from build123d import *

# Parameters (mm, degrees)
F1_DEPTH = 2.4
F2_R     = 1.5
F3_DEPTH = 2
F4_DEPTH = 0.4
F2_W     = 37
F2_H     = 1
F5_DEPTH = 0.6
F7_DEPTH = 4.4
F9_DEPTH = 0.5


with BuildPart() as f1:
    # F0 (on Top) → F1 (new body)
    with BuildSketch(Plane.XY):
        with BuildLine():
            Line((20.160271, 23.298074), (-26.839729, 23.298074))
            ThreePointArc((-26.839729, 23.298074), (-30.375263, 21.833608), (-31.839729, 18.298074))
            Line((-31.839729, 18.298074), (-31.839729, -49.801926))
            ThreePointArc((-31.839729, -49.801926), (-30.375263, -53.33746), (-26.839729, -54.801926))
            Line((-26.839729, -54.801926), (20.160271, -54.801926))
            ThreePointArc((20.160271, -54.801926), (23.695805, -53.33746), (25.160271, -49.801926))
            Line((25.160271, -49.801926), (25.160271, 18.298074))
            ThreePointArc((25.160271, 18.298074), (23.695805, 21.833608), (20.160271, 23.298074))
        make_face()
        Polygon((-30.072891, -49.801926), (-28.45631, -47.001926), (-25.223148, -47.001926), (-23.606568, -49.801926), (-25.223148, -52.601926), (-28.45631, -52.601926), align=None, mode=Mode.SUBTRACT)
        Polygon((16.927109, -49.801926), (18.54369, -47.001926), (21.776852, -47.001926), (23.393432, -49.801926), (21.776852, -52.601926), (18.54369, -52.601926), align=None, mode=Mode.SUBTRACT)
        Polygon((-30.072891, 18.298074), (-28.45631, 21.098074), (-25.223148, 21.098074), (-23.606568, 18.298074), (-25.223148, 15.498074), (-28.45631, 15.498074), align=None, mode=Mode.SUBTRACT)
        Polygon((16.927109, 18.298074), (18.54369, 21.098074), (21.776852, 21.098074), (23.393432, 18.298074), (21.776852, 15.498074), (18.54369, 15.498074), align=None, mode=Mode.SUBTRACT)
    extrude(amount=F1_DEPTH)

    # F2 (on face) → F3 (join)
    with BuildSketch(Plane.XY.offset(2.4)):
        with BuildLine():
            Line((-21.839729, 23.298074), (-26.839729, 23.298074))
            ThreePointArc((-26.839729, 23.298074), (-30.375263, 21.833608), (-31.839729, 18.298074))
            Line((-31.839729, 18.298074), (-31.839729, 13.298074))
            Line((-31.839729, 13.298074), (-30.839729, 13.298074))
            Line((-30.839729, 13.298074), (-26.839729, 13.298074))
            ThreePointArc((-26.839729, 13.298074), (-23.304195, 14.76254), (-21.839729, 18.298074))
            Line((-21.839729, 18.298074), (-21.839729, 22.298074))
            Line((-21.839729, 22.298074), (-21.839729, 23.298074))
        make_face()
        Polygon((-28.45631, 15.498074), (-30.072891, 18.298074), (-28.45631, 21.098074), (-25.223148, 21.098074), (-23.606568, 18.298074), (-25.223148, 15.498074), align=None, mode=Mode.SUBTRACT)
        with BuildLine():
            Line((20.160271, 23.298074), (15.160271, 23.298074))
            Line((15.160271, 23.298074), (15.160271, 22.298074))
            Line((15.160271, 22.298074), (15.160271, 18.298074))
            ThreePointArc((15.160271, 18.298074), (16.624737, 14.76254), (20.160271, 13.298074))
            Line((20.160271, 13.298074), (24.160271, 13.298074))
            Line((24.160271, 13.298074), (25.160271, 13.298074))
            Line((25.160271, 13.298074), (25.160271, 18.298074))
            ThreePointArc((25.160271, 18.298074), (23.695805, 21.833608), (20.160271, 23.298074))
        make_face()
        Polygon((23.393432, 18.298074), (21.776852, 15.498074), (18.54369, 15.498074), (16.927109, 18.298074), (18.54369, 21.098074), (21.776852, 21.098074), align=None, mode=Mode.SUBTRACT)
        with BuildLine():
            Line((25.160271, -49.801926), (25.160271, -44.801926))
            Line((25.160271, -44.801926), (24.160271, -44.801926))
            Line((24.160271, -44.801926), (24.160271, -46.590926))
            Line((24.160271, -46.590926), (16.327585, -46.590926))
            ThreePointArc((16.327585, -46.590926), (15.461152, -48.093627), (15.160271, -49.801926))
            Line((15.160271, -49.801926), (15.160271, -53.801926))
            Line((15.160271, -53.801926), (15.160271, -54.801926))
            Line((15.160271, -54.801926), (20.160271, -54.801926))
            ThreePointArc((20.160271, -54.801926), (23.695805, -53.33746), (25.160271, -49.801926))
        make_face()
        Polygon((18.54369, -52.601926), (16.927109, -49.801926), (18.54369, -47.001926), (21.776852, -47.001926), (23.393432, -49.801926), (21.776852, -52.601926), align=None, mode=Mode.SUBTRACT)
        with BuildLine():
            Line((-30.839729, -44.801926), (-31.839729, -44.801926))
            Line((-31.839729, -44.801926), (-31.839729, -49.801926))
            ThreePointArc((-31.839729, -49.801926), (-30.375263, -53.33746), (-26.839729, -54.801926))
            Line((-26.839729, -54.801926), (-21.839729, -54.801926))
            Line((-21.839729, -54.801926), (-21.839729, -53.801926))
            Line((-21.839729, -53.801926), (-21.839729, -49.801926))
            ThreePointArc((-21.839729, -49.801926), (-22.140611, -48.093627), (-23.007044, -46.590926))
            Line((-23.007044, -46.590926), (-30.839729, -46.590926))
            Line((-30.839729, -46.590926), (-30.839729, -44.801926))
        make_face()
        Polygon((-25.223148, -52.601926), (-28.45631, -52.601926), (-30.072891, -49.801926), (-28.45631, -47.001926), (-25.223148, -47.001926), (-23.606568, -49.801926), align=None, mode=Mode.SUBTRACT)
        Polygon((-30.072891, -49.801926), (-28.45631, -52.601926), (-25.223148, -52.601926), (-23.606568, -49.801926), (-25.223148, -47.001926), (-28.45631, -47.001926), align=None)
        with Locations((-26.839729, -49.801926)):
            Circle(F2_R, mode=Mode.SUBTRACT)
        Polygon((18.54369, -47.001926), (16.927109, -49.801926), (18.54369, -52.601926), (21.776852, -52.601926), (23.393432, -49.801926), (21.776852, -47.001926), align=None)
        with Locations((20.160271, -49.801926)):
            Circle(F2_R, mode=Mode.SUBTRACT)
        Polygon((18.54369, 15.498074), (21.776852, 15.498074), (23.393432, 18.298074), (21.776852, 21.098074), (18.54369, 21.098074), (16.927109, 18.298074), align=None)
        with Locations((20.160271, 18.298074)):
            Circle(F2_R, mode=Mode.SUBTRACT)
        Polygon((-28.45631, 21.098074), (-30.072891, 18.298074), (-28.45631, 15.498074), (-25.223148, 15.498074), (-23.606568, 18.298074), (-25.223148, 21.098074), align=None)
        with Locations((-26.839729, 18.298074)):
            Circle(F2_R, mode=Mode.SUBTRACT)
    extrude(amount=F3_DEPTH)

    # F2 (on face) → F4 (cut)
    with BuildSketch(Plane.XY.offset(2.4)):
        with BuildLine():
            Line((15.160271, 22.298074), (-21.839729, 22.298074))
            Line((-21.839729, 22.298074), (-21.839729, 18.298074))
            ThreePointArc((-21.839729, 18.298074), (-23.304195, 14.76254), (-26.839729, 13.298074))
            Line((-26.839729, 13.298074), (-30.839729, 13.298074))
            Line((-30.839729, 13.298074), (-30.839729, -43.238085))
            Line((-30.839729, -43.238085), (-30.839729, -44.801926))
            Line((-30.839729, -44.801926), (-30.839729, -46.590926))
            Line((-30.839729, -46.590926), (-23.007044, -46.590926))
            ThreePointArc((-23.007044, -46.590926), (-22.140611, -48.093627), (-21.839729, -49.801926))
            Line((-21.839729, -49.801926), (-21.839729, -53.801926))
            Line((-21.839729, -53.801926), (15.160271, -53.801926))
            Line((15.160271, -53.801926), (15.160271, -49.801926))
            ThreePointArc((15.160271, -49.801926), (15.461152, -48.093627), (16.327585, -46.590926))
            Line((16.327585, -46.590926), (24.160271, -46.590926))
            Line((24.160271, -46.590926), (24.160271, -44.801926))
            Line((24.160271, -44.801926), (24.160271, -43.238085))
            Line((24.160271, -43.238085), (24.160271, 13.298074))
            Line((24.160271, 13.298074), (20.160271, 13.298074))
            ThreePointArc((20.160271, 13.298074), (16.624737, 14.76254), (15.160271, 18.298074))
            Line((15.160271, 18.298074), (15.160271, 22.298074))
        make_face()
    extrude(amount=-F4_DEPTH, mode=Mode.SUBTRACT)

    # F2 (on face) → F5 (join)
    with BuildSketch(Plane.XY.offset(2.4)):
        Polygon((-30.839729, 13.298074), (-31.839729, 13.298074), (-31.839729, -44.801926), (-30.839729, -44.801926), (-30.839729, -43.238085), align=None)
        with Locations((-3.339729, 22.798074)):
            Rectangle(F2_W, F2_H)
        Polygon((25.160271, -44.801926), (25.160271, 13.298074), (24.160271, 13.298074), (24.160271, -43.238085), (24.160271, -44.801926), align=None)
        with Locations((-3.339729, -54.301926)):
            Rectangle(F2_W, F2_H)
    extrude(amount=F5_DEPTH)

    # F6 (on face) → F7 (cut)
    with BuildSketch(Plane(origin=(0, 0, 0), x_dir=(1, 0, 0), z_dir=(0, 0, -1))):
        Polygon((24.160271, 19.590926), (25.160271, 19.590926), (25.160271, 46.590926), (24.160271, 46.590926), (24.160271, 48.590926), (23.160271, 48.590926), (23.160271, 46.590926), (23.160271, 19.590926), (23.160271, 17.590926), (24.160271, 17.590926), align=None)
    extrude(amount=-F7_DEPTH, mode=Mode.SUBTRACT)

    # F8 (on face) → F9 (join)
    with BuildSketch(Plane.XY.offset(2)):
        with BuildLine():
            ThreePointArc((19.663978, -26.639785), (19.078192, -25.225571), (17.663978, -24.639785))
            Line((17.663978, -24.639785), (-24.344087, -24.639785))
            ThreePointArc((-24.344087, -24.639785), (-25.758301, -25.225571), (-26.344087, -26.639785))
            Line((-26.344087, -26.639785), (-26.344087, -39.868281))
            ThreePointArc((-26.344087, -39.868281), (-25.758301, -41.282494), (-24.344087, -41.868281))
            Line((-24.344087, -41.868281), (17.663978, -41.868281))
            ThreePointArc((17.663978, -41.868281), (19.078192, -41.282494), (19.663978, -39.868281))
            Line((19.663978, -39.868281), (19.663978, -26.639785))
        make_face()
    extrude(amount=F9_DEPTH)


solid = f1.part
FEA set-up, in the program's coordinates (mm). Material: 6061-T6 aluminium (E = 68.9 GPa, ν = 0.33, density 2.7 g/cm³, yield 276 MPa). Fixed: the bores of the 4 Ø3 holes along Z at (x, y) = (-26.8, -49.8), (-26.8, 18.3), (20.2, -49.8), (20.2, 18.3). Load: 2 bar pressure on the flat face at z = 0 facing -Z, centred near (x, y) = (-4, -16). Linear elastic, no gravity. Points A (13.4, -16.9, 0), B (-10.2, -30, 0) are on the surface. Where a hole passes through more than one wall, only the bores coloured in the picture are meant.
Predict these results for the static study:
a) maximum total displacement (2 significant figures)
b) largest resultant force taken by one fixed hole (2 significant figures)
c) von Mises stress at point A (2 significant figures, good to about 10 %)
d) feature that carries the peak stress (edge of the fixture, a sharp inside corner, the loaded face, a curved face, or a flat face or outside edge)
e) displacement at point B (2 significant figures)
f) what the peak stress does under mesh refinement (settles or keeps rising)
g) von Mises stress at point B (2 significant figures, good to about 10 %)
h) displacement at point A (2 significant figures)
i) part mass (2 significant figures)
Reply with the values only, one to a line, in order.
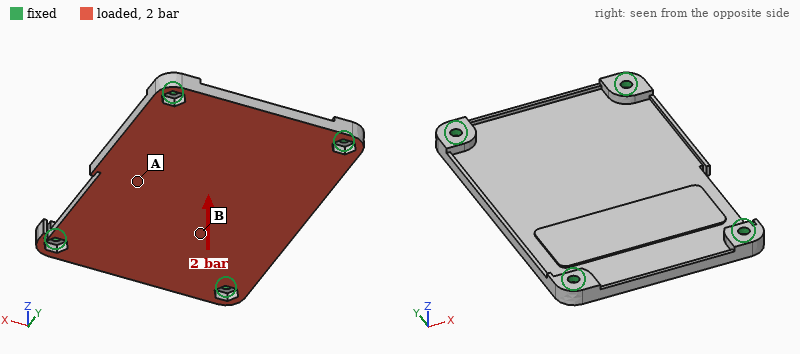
0.28 mm
500 N
64 MPa
edge of the fixture
0.20 mm
keeps rising
30 MPa
0.26 mm
26 g
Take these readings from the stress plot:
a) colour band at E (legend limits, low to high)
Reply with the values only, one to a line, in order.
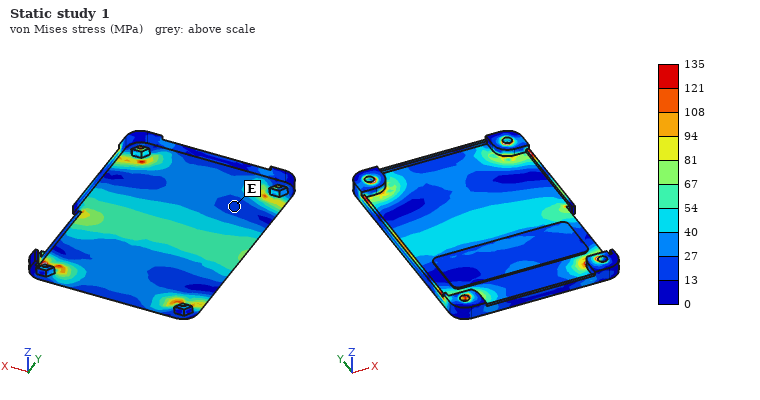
13 to 27 MPa
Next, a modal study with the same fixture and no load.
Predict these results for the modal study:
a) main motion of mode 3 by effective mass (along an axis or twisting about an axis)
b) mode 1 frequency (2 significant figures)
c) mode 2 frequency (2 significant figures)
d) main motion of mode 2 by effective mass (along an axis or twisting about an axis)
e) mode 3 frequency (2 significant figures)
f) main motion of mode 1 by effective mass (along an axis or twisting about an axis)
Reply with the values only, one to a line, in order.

twisting about X
2100 Hz
3300 Hz
twisting about Y
5100 Hz
along Z
